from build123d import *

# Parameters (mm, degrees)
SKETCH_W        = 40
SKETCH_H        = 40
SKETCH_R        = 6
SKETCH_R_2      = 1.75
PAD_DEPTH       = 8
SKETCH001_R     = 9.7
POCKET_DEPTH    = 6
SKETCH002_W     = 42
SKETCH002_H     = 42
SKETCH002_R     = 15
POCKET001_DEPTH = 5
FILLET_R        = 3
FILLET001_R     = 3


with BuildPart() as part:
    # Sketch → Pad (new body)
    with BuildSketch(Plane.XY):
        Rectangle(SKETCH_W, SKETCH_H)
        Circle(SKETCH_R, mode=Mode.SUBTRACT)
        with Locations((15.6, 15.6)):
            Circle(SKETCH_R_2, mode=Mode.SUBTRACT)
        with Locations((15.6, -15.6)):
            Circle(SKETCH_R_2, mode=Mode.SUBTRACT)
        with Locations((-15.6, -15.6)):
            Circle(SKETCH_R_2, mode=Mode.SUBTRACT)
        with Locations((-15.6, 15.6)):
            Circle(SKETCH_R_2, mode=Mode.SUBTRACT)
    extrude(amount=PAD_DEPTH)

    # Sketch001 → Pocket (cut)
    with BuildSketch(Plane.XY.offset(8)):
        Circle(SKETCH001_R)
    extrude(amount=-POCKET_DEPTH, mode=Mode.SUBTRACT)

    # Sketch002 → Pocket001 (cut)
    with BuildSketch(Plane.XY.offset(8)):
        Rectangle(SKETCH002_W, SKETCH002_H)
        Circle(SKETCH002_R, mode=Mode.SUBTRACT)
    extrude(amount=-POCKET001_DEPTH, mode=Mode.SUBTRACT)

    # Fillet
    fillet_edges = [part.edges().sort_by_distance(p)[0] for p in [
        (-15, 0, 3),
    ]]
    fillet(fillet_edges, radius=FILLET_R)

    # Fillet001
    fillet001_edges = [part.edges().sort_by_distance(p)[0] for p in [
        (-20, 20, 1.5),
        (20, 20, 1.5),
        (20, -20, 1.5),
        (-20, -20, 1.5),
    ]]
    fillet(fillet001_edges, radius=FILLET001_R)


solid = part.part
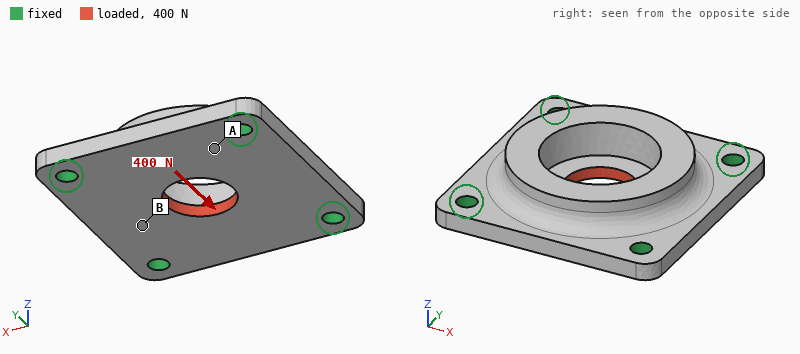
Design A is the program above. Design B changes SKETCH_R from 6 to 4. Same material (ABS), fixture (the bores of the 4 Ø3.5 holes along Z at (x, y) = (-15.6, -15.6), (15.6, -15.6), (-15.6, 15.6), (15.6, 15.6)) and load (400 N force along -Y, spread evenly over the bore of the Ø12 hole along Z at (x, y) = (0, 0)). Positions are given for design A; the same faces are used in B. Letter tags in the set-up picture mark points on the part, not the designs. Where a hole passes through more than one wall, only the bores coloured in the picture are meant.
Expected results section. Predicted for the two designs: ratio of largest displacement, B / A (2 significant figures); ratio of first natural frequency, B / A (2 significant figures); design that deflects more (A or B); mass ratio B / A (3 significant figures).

1.1
0.98
B
1.02
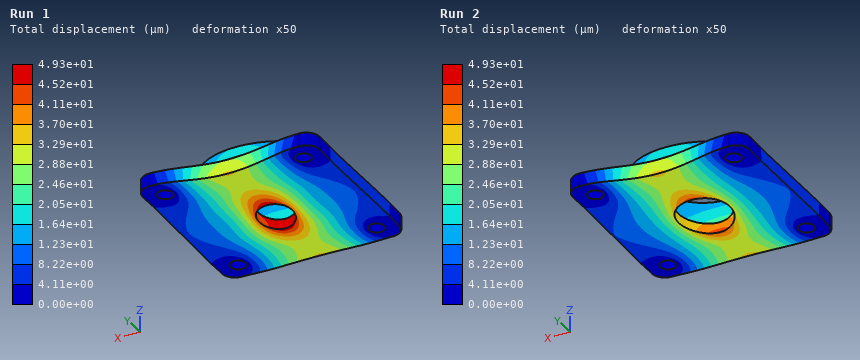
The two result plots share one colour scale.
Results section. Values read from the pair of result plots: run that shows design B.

Run 1
